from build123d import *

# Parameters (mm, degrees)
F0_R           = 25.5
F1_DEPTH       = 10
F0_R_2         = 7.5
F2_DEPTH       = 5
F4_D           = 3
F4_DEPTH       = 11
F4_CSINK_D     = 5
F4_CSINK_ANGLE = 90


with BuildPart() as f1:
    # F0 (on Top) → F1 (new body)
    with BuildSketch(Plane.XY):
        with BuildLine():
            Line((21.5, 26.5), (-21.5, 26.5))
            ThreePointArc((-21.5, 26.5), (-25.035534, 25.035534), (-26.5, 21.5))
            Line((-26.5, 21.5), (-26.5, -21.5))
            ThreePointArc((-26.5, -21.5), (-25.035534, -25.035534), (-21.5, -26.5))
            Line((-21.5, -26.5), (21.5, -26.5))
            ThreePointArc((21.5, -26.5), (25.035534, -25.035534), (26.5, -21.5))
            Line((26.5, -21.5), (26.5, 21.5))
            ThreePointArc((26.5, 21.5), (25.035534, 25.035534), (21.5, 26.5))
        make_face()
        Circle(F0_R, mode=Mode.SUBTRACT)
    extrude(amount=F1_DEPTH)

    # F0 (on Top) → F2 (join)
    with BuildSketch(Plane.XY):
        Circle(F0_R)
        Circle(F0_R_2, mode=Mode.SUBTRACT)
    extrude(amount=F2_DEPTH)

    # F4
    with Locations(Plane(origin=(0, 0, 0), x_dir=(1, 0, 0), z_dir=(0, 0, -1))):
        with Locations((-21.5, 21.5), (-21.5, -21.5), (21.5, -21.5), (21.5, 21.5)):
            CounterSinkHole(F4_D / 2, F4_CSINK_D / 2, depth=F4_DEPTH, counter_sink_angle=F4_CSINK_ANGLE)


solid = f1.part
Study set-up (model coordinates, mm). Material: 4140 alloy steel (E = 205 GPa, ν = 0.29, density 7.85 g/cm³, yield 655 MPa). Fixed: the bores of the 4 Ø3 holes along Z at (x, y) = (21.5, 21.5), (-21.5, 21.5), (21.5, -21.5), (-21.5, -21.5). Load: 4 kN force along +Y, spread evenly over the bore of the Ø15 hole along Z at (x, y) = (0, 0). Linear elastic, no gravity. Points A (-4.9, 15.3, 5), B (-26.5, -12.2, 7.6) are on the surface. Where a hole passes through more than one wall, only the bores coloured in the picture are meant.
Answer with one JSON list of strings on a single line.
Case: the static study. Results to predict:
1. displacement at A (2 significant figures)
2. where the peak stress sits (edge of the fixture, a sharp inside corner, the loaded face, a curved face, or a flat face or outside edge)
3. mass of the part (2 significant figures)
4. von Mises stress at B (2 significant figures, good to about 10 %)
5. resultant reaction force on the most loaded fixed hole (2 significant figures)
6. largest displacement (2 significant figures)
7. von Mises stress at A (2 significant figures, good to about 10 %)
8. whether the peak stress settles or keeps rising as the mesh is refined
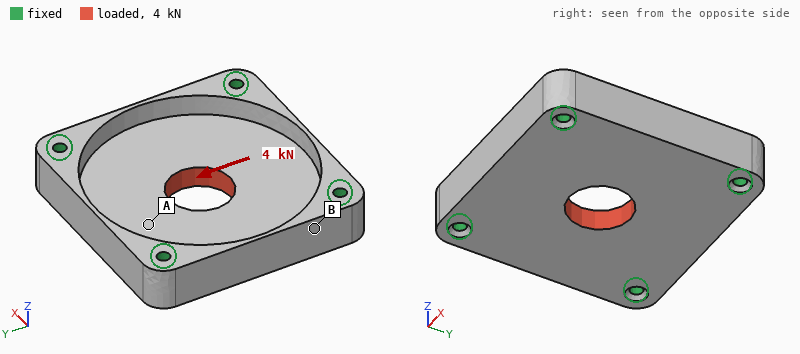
["2.0 µm", "edge of the fixture", "130 g", "5.3 MPa", "1.1 kN", "2.6 µm", "12 MPa", "keeps rising"]
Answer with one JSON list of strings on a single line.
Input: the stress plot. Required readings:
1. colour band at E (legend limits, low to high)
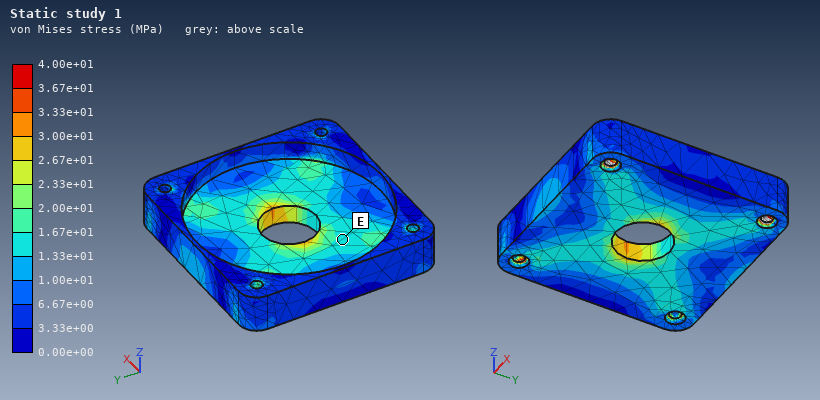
["1.33e+01 to 1.67e+01 MPa"]
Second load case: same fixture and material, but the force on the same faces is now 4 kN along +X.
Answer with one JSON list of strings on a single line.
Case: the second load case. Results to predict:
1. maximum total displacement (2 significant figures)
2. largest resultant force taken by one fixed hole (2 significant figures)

["2.6 µm", "1.1 kN"]
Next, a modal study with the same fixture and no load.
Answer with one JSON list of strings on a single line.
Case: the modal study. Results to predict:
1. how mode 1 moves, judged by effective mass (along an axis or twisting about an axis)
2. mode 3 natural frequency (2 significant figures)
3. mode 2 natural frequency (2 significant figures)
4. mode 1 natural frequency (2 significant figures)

["along Z", "19 kHz", "19 kHz", "12 kHz"]
